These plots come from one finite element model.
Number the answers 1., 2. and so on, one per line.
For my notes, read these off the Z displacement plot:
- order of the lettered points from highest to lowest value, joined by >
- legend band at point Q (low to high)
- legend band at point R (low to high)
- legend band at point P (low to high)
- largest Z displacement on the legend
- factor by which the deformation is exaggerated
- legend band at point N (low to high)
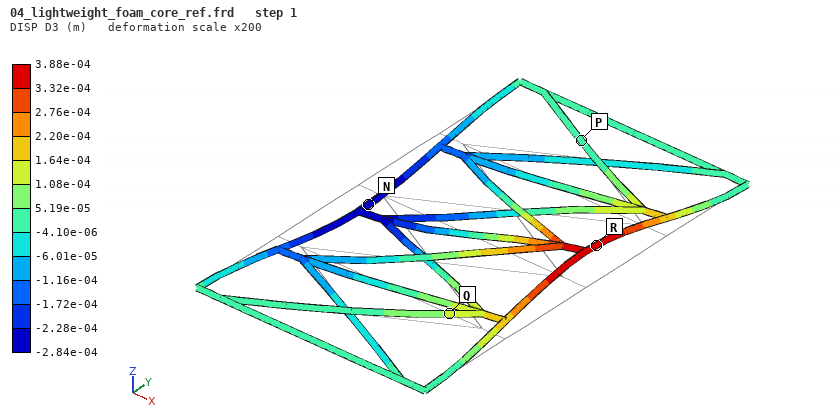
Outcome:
1. R > Q > P > N
2. 1.08e-04 to 1.64e-04 m
3. 3.32e-04 to 3.88e-04 m
4. -4.10e-06 to 5.19e-05 m
5. 3.88e-04 m
6. 200
7. -2.84e-04 to -2.28e-04 m
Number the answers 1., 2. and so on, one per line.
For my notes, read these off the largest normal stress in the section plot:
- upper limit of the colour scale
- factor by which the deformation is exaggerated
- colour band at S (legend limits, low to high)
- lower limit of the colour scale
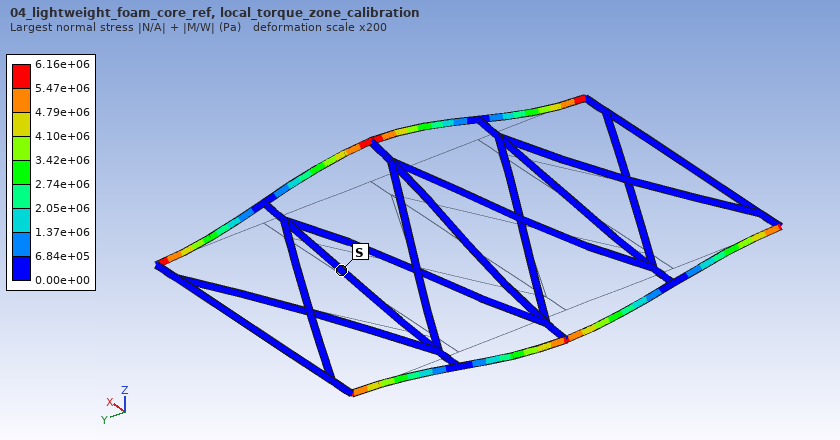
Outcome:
1. 6.16e+06 Pa
2. 200
3. 0.00e+00 to 6.84e+05 Pa
4. 0.00e+00 Pa
